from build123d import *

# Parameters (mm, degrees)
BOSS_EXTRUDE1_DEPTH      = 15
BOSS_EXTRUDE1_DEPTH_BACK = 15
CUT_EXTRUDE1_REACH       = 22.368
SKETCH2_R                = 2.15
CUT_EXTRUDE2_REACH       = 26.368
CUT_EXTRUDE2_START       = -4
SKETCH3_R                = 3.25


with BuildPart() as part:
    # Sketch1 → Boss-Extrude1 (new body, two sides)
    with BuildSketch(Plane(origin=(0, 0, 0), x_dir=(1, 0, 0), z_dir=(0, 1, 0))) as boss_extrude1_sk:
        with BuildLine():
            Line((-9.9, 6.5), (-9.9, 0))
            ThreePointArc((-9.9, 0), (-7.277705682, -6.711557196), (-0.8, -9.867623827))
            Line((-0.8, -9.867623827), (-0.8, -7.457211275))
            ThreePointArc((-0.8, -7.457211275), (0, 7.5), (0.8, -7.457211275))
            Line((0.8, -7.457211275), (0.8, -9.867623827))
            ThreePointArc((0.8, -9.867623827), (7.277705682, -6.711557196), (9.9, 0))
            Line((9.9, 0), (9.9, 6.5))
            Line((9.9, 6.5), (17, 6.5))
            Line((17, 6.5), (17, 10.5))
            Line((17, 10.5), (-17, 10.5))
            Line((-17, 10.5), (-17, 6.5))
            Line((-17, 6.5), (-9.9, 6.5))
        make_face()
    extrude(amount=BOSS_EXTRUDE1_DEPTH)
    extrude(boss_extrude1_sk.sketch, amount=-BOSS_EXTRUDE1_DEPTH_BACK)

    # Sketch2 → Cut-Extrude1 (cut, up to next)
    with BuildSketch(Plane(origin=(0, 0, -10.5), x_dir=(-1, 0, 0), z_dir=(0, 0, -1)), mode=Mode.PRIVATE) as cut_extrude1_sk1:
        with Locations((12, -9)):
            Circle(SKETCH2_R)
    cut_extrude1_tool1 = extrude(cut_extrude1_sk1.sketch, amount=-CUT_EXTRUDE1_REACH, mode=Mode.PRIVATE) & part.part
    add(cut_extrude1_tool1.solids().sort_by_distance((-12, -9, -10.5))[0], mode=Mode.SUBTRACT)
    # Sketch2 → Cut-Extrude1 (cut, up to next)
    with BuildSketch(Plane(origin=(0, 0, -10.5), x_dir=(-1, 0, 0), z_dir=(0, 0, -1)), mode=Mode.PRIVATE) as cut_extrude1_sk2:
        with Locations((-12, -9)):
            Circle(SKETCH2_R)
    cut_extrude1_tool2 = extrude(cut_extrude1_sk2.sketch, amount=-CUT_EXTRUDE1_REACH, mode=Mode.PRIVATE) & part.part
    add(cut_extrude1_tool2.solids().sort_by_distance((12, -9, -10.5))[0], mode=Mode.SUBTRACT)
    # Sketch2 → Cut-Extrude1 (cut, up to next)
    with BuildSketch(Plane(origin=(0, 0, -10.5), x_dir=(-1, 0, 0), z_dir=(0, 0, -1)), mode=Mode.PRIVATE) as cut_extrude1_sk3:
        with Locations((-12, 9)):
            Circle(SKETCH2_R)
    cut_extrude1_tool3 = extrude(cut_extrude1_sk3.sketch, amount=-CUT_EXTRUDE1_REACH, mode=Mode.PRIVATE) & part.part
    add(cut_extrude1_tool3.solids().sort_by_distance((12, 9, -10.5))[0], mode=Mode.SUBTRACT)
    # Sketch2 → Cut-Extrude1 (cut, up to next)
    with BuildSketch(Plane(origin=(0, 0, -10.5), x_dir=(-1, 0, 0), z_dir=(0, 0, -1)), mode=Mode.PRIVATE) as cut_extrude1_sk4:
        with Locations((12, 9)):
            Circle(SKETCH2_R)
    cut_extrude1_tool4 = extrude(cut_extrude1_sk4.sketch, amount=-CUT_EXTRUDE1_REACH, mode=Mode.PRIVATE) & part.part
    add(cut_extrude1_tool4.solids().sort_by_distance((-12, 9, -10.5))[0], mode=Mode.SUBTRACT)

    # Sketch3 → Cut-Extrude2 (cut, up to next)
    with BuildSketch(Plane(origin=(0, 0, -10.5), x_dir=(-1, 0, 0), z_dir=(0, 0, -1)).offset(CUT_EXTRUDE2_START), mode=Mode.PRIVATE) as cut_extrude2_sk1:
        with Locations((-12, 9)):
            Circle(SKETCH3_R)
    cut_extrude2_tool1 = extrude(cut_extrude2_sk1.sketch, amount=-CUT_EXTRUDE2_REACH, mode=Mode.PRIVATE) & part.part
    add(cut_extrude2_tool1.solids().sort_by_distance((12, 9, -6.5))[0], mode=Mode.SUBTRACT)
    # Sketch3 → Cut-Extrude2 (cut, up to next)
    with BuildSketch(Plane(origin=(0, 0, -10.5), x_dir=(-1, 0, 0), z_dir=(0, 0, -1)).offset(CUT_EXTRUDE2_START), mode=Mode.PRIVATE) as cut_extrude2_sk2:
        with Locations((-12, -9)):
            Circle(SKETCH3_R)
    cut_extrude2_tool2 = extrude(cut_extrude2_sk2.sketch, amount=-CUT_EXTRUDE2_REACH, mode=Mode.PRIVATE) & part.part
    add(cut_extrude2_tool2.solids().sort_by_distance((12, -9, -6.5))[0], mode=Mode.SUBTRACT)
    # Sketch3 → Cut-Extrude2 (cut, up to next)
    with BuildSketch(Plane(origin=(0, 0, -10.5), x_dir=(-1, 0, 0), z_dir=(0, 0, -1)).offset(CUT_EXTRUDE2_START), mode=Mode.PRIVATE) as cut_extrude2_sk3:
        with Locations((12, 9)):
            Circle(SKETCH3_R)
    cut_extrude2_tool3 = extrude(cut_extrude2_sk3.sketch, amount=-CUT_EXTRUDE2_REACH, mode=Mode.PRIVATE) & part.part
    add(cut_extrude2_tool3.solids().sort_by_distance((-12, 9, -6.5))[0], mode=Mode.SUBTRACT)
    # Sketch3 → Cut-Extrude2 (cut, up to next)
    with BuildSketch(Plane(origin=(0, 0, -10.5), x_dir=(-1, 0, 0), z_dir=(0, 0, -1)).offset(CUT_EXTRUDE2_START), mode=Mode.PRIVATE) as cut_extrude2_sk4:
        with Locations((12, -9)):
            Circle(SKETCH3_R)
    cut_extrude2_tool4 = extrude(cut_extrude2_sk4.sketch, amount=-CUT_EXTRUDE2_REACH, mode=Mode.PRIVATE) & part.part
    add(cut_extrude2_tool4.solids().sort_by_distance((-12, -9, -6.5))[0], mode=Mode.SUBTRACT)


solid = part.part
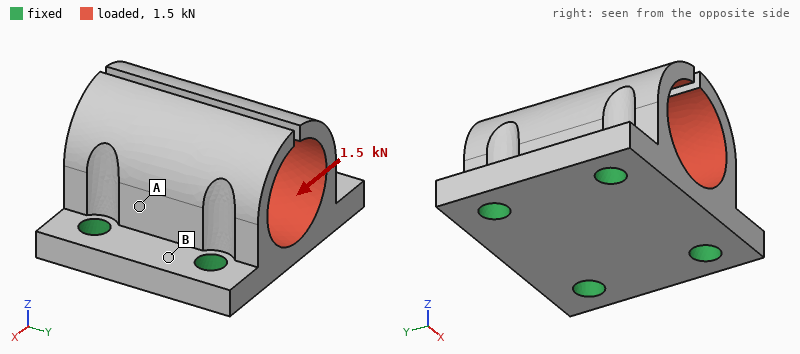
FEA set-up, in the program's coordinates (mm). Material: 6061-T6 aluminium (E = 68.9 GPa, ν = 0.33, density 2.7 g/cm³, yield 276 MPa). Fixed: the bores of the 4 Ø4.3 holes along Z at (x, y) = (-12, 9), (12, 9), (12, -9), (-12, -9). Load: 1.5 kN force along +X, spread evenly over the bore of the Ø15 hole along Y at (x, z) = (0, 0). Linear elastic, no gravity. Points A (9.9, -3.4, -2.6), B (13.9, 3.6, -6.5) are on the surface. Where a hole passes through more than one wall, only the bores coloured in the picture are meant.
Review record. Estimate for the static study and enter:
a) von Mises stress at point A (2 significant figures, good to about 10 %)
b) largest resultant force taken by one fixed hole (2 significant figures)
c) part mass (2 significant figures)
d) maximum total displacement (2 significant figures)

71 MPa
450 N
18 g
98 µm
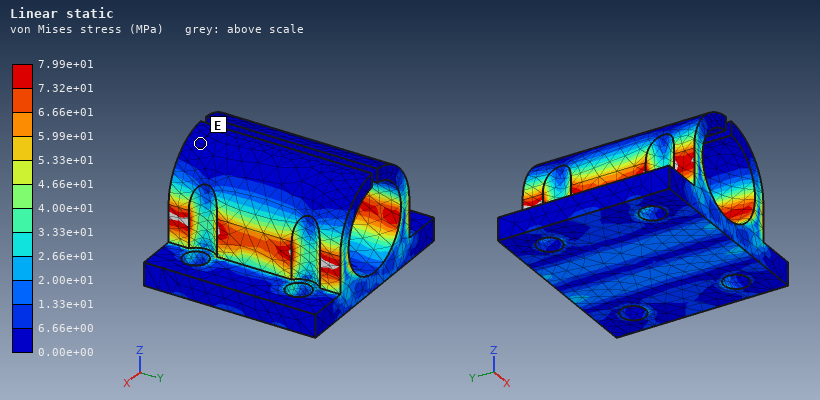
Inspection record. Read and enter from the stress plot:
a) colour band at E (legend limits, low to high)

0.00e+00 to 6.66e+00 MPa
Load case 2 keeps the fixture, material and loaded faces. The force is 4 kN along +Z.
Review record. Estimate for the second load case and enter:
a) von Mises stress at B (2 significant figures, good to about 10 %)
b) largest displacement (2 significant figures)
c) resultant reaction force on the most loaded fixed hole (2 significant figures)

23 MPa
0.21 mm
1.0 kN
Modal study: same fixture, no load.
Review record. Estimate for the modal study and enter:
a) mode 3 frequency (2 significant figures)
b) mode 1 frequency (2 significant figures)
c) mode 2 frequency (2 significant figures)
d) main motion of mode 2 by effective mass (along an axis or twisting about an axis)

10 kHz
6300 Hz
6800 Hz
along X
